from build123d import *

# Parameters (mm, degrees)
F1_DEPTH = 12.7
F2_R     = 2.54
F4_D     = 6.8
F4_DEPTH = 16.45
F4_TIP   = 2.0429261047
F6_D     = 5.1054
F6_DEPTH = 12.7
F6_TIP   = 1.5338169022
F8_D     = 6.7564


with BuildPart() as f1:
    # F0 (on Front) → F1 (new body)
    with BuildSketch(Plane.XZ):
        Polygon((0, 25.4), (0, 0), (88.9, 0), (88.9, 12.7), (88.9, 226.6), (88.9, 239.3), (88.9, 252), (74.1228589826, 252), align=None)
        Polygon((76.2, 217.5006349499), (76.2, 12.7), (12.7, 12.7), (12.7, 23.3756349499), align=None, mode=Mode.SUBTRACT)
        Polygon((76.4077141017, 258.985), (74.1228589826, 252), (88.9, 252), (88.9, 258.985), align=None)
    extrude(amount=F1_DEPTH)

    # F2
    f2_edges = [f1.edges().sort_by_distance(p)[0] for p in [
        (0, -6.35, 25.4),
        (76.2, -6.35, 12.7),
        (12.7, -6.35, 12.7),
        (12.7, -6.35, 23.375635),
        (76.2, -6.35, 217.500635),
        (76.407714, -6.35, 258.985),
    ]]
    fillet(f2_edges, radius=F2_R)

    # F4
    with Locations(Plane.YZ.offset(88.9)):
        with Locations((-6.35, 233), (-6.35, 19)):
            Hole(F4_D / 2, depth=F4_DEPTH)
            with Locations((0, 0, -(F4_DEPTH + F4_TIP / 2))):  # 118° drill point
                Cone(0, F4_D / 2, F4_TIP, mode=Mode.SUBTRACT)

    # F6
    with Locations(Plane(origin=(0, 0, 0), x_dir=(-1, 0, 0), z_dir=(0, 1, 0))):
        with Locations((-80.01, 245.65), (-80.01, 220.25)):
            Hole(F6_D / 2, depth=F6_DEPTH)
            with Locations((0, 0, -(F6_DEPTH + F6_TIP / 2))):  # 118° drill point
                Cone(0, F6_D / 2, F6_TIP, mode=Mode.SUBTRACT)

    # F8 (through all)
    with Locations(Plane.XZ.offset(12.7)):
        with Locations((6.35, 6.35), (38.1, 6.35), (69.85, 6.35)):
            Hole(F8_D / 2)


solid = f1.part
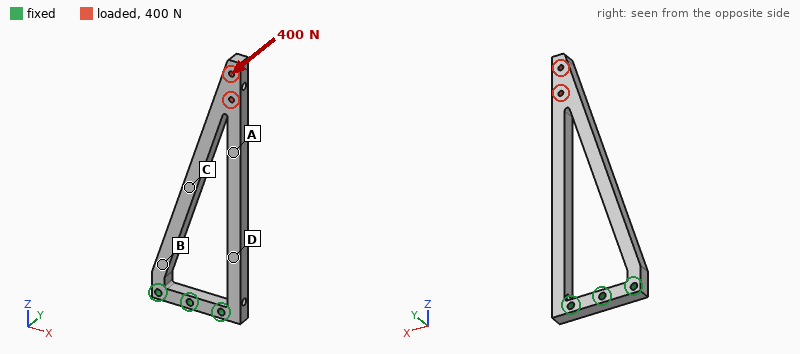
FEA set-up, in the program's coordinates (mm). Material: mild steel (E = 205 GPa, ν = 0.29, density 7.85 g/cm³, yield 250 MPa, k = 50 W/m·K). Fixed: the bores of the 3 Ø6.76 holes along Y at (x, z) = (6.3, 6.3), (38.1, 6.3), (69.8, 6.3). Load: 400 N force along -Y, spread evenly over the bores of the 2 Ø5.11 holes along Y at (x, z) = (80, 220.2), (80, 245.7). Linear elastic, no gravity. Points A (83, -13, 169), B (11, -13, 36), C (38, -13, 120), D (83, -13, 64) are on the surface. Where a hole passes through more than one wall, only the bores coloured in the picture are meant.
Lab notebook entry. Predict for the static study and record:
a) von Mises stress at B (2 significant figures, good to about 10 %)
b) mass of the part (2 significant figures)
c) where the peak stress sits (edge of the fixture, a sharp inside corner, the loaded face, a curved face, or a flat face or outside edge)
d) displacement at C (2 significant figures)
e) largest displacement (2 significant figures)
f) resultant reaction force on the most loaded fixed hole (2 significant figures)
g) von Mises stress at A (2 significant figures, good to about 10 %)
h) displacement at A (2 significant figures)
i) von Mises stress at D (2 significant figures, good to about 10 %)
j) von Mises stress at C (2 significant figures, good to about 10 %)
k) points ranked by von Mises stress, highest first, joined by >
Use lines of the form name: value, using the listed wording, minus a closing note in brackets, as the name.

von Mises stress at B: 120 MPa
mass of the part: 700 g
where the peak stress sits: a curved face
displacement at C: 0.59 mm
largest displacement: 2.3 mm
resultant reaction force on the most loaded fixed hole: 220 N
von Mises stress at A: 35 MPa
displacement at A: 1.2 mm
von Mises stress at D: 97 MPa
von Mises stress at C: 68 MPa
points ranked by von Mises stress, highest first, joined by >: B > D > C > A
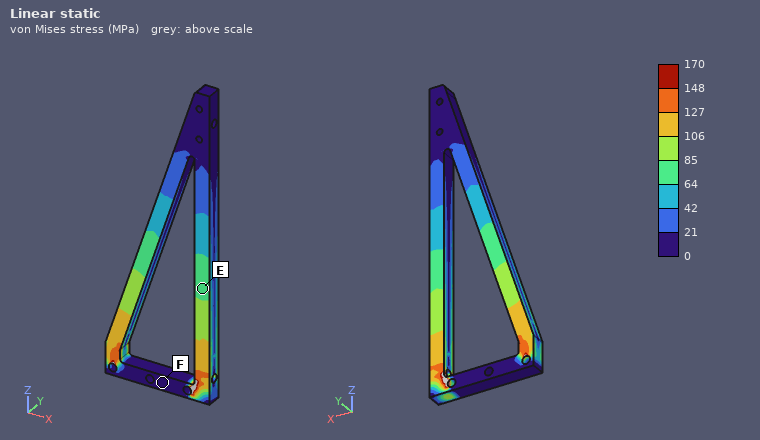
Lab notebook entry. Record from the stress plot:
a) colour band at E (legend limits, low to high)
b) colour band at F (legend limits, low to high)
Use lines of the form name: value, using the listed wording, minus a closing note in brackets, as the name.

colour band at E: 64 to 85 MPa
colour band at F: 0 to 21 MPa
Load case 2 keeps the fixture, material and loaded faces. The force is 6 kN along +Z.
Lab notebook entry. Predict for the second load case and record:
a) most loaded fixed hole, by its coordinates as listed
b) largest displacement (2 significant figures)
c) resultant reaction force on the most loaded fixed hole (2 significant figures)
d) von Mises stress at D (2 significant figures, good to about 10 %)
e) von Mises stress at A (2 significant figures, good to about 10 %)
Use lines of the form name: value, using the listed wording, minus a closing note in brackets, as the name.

most loaded fixed hole, by its coordinates as listed: (69.8, 6.3)
largest displacement: 0.16 mm
resultant reaction force on the most loaded fixed hole: 6.0 kN
von Mises stress at D: 36 MPa
von Mises stress at A: 36 MPa
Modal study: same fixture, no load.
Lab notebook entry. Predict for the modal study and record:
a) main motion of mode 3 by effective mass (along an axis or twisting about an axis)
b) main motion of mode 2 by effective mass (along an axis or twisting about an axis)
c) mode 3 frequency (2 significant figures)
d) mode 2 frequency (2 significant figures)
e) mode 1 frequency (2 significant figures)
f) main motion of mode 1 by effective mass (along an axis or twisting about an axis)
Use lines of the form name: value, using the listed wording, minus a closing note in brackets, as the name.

main motion of mode 3 by effective mass: along Y
main motion of mode 2 by effective mass: along X
mode 3 frequency: 1000 Hz
mode 2 frequency: 590 Hz
mode 1 frequency: 170 Hz
main motion of mode 1 by effective mass: along Y
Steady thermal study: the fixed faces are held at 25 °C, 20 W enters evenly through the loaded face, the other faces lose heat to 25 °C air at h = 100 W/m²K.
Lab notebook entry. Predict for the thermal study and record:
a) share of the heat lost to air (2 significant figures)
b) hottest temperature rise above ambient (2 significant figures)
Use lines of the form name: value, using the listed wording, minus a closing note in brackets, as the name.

share of the heat lost to air: 100 %
hottest temperature rise above ambient: 39 K
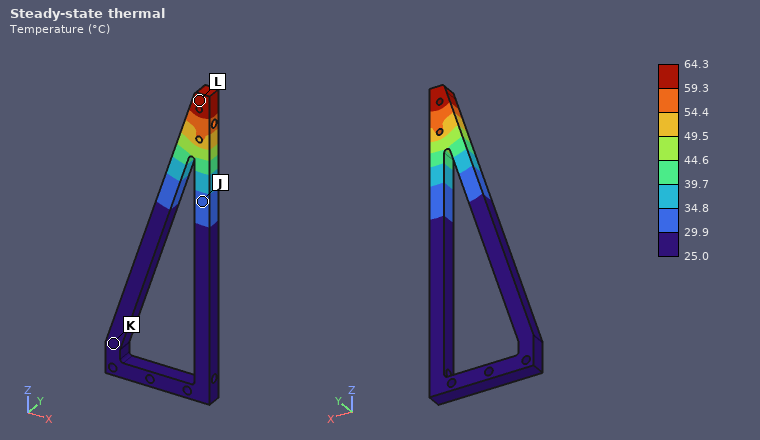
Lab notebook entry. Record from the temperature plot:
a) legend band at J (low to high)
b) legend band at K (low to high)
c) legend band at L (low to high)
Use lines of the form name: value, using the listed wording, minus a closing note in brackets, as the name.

legend band at J: 29.9 to 34.8 °C
legend band at K: 25.0 to 29.9 °C
legend band at L: 59.3 to 64.3 °C
